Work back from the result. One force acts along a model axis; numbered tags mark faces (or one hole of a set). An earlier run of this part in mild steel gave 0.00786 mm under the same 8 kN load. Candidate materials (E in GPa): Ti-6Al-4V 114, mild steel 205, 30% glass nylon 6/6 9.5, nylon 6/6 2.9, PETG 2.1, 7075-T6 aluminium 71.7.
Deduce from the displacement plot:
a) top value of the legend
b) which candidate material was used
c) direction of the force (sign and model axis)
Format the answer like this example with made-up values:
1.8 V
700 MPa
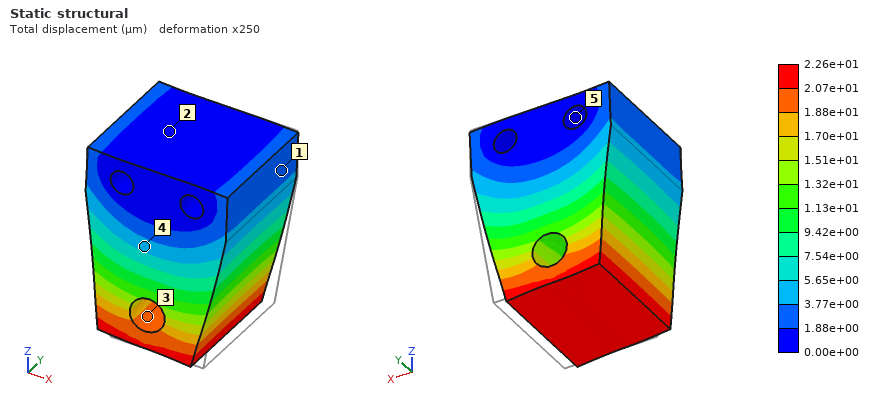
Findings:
2.26e+01 µm
7075-T6 aluminium
-X
